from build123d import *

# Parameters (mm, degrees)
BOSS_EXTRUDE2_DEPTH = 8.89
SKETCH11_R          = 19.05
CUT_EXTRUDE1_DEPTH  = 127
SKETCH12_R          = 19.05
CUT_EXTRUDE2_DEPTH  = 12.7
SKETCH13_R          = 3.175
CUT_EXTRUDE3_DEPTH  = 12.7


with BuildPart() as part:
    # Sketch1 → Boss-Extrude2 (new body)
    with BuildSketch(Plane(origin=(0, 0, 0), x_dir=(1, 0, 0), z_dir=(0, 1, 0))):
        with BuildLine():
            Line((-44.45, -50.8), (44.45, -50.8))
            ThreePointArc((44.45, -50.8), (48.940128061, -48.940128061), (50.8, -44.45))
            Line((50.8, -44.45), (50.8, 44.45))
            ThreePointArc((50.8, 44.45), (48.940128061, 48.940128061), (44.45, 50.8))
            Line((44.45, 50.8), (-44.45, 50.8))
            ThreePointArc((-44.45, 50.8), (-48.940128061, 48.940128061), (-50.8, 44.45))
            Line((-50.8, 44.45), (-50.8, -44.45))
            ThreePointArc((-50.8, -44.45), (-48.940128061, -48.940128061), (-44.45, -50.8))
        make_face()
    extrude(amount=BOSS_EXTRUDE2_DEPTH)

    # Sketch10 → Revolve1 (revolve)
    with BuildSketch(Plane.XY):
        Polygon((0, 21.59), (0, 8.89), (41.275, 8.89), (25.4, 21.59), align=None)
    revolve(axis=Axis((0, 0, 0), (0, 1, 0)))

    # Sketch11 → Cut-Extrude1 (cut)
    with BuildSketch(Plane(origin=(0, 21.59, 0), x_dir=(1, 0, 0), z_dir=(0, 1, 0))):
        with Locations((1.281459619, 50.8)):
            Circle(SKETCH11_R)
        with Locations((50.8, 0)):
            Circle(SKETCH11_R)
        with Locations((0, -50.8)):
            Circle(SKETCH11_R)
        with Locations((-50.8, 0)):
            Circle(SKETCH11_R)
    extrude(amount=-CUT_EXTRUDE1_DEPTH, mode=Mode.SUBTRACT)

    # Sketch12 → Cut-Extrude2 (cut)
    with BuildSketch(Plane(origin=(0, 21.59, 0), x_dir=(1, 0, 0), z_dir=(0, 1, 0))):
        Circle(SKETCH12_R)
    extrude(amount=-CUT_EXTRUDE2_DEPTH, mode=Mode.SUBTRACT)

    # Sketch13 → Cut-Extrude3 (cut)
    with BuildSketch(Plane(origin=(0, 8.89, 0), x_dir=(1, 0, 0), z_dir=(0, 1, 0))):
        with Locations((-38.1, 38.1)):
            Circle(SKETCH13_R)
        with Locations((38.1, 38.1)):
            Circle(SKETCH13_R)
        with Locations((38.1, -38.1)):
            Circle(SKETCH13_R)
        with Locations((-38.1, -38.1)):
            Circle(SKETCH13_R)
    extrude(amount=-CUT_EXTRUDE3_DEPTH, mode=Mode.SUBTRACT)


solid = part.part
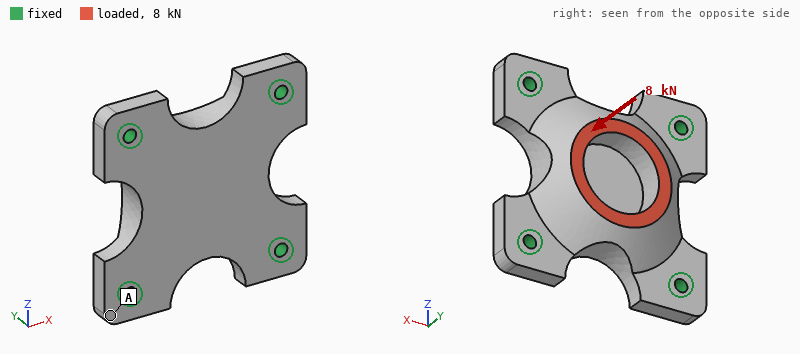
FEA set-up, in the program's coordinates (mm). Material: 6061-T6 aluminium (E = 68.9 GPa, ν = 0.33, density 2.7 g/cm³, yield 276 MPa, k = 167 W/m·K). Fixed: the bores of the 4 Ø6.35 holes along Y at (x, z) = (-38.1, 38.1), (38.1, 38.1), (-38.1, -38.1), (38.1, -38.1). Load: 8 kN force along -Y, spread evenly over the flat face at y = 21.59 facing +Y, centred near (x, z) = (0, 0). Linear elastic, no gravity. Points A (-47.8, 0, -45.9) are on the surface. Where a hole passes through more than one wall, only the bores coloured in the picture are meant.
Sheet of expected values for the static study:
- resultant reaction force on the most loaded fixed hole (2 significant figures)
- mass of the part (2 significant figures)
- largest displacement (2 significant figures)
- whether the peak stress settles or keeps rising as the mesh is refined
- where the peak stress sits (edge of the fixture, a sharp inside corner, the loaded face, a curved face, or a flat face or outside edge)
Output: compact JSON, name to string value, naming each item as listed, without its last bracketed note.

{"resultant reaction force on the most loaded fixed hole": "2.5 kN", "mass of the part": "270 g", "largest displacement": "36 µm", "whether the peak stress settles or keeps rising as the mesh is refined": "keeps rising", "where the peak stress sits": "edge of the fixture"}
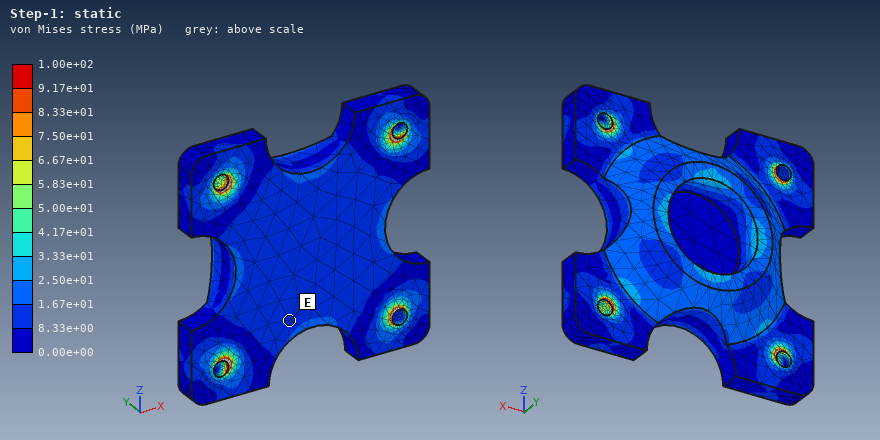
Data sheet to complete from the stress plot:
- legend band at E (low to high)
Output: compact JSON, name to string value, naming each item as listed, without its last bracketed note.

{"legend band at E": "8.33e+00 to 1.67e+01 MPa"}
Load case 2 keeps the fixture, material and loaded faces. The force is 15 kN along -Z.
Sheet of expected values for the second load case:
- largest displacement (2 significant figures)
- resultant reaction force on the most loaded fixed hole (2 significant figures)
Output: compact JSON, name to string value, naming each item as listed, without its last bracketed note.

{"largest displacement": "32 µm", "resultant reaction force on the most loaded fixed hole": "4.9 kN"}
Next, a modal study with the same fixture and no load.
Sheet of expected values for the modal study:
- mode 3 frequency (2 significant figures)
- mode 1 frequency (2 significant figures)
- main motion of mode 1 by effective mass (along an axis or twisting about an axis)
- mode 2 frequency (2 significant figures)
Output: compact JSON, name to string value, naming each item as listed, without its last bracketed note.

{"mode 3 frequency": "10 kHz", "mode 1 frequency": "6200 Hz", "main motion of mode 1 by effective mass": "along Y", "mode 2 frequency": "10 kHz"}
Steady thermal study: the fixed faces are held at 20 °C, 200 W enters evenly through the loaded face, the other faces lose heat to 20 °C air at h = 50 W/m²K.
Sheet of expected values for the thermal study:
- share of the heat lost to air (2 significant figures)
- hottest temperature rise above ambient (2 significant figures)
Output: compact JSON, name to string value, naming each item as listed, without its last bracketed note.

{"share of the heat lost to air": "8.9 %", "hottest temperature rise above ambient": "35 K"}
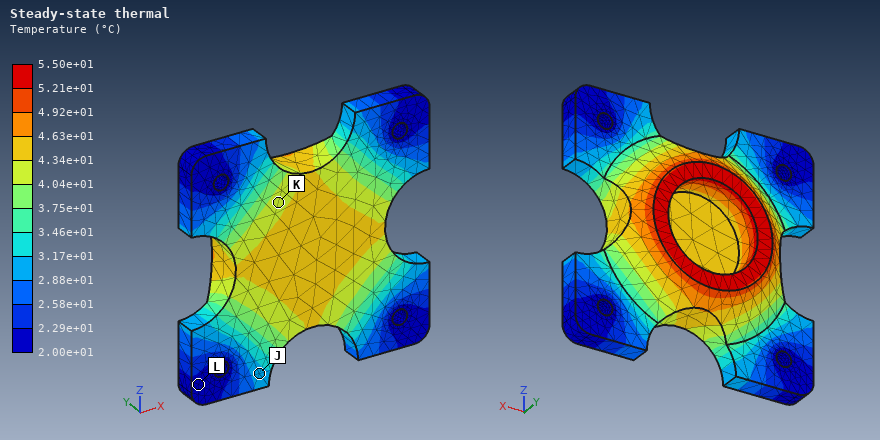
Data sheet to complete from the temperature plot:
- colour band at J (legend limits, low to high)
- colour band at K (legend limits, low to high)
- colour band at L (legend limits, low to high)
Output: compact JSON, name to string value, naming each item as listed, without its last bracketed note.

{"colour band at J": "2.88e+01 to 3.17e+01 °C", "colour band at K": "4.04e+01 to 4.34e+01 °C", "colour band at L": "2.00e+01 to 2.29e+01 °C"}
